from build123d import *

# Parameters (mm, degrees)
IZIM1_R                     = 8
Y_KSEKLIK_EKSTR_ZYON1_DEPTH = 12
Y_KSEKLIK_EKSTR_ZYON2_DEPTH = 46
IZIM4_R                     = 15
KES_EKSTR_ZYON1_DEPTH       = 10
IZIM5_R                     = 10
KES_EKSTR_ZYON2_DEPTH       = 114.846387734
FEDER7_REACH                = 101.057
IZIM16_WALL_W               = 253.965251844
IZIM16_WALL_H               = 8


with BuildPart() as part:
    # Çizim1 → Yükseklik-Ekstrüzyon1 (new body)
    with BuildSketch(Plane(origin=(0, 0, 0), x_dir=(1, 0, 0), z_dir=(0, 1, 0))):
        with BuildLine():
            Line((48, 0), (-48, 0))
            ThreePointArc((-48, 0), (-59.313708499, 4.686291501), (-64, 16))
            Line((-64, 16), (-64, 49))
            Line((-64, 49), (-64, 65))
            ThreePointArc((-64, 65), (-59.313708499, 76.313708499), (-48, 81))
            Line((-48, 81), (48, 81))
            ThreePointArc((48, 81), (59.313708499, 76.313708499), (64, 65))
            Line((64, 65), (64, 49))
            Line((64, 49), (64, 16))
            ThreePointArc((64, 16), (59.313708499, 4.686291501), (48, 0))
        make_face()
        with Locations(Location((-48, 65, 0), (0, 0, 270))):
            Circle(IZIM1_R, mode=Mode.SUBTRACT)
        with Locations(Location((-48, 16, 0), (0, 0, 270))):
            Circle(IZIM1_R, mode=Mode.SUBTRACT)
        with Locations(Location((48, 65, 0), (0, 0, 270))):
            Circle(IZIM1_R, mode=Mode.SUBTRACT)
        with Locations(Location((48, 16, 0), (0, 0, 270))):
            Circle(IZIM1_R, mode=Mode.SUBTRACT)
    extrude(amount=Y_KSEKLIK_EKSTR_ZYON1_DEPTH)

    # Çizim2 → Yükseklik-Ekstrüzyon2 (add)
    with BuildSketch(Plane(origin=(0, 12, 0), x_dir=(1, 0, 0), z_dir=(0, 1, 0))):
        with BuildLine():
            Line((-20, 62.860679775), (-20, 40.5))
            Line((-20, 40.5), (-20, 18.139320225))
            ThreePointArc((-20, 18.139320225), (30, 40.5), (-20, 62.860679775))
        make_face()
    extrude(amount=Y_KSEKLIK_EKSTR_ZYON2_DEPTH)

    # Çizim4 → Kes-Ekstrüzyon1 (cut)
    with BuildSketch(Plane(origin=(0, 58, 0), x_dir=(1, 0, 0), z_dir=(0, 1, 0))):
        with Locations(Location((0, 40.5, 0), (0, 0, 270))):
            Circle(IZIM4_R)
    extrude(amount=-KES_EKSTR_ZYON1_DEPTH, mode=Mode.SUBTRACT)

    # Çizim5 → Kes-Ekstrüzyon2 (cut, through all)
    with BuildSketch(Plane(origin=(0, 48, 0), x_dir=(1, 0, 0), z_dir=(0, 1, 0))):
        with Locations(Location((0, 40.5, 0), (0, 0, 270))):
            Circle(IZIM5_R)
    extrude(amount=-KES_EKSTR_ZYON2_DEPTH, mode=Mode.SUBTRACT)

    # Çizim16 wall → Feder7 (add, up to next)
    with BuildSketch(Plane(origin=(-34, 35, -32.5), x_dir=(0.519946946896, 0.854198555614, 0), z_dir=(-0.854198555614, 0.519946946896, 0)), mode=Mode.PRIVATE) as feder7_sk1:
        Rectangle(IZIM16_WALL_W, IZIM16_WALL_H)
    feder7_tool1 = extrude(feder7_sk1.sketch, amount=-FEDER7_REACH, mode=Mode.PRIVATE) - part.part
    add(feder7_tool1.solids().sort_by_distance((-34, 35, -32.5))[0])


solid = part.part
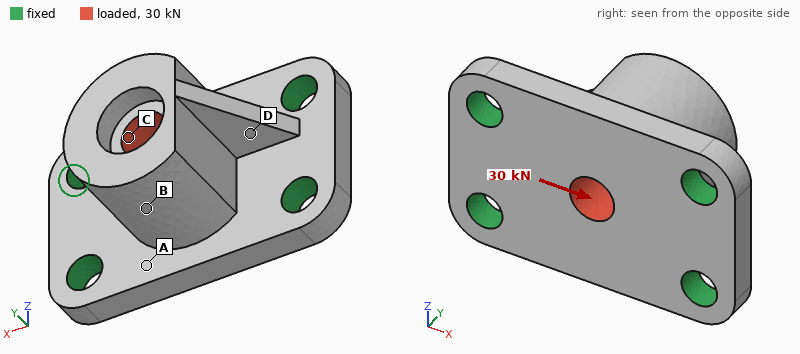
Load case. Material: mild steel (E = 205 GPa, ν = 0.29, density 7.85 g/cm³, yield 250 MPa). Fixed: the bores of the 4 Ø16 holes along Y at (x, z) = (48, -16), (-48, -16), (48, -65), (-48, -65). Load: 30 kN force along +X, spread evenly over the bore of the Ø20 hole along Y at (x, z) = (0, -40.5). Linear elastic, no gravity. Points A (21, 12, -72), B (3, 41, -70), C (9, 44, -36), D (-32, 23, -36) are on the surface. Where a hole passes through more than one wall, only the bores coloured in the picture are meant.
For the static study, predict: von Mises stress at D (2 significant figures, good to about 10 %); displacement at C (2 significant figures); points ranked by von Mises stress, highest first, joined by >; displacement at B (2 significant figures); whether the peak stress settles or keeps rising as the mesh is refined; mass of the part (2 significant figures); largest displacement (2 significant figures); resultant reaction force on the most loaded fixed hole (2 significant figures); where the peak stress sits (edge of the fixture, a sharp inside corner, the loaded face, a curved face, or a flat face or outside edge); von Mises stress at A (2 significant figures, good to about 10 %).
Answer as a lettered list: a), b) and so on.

a) 34 MPa
b) 13 µm
c) D > A > C > B
d) 11 µm
e) keeps rising
f) 1.7 kg
g) 17 µm
h) 9.6 kN
i) edge of the fixture
j) 23 MPa
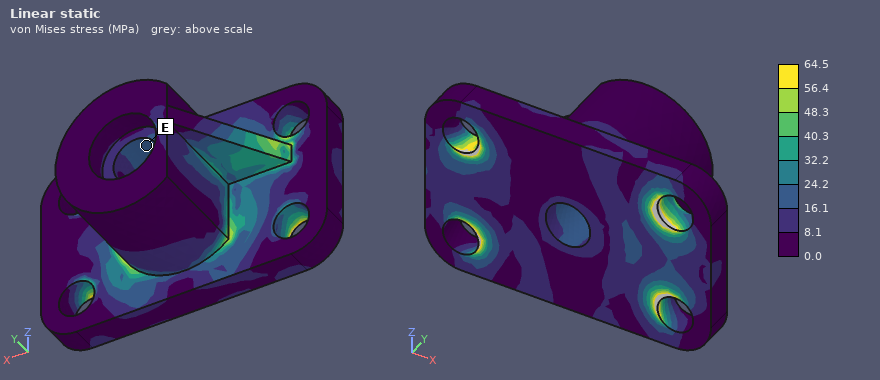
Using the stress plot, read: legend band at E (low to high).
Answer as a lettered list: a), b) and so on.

a) 16.1 to 24.2 MPa
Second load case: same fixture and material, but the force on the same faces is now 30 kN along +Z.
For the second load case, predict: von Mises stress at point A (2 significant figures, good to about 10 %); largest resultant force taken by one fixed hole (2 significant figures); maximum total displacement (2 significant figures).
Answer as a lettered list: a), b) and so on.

a) 43 MPa
b) 11 kN
c) 45 µm
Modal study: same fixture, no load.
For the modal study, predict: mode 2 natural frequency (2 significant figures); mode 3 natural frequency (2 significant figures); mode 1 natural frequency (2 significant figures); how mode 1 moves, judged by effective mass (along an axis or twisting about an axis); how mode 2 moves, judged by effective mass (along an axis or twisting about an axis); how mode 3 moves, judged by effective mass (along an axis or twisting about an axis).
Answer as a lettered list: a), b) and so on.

a) 6100 Hz
b) 7100 Hz
c) 4100 Hz
d) along Z
e) along Y
f) along X
